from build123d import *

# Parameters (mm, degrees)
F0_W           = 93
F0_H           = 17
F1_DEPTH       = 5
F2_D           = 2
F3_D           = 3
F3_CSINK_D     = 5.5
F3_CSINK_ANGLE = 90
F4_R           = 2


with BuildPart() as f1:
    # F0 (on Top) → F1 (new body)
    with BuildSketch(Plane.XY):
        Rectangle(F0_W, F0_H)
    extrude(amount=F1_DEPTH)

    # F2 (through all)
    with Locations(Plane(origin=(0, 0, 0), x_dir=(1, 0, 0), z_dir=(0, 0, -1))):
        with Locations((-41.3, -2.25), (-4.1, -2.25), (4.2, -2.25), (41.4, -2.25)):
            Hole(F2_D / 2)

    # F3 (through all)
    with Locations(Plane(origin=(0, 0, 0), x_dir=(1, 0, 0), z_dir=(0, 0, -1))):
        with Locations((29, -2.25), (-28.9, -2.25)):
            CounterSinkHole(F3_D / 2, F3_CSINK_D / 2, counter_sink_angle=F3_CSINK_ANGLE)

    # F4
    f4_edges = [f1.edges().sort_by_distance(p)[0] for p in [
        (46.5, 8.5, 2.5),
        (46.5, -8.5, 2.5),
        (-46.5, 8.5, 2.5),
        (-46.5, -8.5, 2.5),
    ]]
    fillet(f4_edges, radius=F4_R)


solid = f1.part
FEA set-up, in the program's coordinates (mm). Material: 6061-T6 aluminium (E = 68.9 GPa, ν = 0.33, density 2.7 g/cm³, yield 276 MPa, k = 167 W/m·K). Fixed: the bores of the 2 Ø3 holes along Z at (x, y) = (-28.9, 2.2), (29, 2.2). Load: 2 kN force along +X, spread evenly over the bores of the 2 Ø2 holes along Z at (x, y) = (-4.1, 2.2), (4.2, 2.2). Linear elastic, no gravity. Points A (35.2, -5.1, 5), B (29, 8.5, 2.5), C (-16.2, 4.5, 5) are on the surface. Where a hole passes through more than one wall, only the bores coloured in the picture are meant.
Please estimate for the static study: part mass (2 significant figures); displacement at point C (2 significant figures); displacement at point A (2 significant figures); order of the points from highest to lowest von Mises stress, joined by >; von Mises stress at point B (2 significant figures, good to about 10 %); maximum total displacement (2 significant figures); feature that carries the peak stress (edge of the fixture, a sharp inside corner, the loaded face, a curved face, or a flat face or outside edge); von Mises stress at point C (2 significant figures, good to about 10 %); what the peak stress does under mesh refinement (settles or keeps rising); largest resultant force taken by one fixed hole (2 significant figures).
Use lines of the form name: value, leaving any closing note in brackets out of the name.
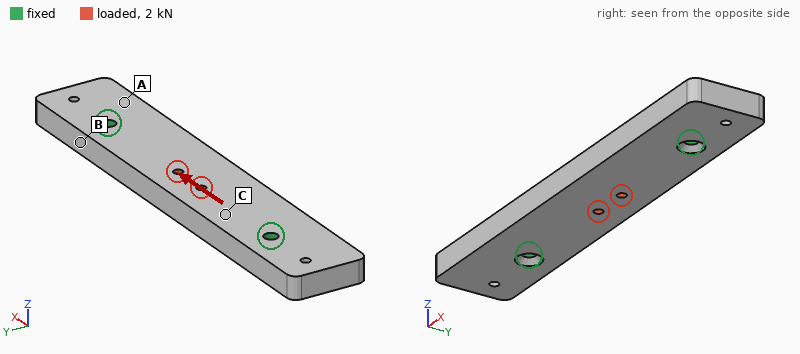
part mass: 21 g
displacement at point C: 3.5 µm
displacement at point A: 2.3 µm
order of the points from highest to lowest von Mises stress, joined by >: C > B > A
von Mises stress at point B: 9.6 MPa
maximum total displacement: 7.6 µm
feature that carries the peak stress: edge of the fixture
von Mises stress at point C: 18 MPa
what the peak stress does under mesh refinement: keeps rising
largest resultant force taken by one fixed hole: 1.0 kN
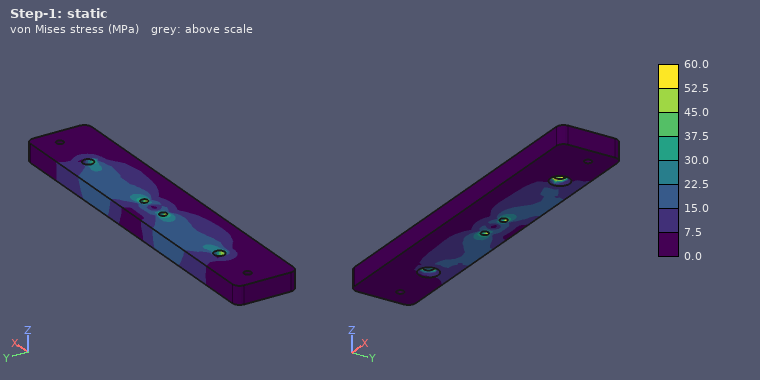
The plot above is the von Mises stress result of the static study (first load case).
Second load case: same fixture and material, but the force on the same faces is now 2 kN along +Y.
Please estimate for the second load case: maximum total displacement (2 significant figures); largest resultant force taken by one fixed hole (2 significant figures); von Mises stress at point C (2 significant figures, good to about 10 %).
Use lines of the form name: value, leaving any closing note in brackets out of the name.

maximum total displacement: 50 µm
largest resultant force taken by one fixed hole: 1.2 kN
von Mises stress at point C: 22 MPa
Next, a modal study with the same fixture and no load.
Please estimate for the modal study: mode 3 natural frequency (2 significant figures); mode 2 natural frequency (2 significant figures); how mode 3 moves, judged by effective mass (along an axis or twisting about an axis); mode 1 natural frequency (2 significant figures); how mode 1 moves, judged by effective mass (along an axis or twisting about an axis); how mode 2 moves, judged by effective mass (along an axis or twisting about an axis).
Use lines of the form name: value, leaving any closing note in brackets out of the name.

mode 3 natural frequency: 11 kHz
mode 2 natural frequency: 10 kHz
how mode 3 moves, judged by effective mass: along Z
mode 1 natural frequency: 6200 Hz
how mode 1 moves, judged by effective mass: along Z
how mode 2 moves, judged by effective mass: twisting about Y
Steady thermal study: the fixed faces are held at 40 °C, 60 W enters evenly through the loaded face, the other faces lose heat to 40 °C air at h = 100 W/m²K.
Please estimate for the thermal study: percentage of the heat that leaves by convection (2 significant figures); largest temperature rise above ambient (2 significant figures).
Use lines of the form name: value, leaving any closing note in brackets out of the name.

percentage of the heat that leaves by convection: 14 %
largest temperature rise above ambient: 61 K
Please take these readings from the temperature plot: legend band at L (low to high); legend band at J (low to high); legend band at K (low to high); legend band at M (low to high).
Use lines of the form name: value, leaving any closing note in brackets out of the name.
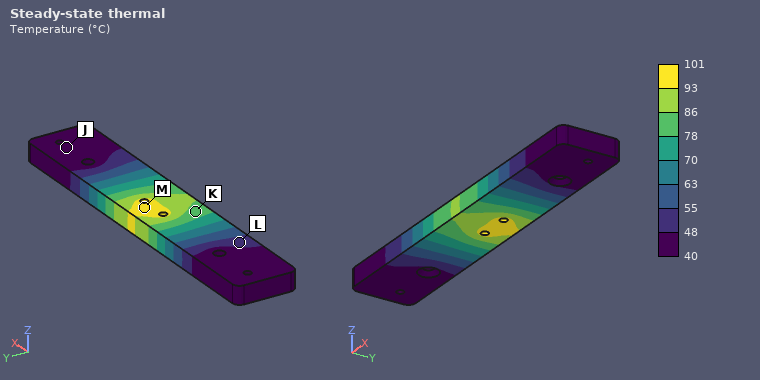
legend band at L: 48 to 55 °C
legend band at J: 40 to 48 °C
legend band at K: 78 to 86 °C
legend band at M: 93 to 101 °C
